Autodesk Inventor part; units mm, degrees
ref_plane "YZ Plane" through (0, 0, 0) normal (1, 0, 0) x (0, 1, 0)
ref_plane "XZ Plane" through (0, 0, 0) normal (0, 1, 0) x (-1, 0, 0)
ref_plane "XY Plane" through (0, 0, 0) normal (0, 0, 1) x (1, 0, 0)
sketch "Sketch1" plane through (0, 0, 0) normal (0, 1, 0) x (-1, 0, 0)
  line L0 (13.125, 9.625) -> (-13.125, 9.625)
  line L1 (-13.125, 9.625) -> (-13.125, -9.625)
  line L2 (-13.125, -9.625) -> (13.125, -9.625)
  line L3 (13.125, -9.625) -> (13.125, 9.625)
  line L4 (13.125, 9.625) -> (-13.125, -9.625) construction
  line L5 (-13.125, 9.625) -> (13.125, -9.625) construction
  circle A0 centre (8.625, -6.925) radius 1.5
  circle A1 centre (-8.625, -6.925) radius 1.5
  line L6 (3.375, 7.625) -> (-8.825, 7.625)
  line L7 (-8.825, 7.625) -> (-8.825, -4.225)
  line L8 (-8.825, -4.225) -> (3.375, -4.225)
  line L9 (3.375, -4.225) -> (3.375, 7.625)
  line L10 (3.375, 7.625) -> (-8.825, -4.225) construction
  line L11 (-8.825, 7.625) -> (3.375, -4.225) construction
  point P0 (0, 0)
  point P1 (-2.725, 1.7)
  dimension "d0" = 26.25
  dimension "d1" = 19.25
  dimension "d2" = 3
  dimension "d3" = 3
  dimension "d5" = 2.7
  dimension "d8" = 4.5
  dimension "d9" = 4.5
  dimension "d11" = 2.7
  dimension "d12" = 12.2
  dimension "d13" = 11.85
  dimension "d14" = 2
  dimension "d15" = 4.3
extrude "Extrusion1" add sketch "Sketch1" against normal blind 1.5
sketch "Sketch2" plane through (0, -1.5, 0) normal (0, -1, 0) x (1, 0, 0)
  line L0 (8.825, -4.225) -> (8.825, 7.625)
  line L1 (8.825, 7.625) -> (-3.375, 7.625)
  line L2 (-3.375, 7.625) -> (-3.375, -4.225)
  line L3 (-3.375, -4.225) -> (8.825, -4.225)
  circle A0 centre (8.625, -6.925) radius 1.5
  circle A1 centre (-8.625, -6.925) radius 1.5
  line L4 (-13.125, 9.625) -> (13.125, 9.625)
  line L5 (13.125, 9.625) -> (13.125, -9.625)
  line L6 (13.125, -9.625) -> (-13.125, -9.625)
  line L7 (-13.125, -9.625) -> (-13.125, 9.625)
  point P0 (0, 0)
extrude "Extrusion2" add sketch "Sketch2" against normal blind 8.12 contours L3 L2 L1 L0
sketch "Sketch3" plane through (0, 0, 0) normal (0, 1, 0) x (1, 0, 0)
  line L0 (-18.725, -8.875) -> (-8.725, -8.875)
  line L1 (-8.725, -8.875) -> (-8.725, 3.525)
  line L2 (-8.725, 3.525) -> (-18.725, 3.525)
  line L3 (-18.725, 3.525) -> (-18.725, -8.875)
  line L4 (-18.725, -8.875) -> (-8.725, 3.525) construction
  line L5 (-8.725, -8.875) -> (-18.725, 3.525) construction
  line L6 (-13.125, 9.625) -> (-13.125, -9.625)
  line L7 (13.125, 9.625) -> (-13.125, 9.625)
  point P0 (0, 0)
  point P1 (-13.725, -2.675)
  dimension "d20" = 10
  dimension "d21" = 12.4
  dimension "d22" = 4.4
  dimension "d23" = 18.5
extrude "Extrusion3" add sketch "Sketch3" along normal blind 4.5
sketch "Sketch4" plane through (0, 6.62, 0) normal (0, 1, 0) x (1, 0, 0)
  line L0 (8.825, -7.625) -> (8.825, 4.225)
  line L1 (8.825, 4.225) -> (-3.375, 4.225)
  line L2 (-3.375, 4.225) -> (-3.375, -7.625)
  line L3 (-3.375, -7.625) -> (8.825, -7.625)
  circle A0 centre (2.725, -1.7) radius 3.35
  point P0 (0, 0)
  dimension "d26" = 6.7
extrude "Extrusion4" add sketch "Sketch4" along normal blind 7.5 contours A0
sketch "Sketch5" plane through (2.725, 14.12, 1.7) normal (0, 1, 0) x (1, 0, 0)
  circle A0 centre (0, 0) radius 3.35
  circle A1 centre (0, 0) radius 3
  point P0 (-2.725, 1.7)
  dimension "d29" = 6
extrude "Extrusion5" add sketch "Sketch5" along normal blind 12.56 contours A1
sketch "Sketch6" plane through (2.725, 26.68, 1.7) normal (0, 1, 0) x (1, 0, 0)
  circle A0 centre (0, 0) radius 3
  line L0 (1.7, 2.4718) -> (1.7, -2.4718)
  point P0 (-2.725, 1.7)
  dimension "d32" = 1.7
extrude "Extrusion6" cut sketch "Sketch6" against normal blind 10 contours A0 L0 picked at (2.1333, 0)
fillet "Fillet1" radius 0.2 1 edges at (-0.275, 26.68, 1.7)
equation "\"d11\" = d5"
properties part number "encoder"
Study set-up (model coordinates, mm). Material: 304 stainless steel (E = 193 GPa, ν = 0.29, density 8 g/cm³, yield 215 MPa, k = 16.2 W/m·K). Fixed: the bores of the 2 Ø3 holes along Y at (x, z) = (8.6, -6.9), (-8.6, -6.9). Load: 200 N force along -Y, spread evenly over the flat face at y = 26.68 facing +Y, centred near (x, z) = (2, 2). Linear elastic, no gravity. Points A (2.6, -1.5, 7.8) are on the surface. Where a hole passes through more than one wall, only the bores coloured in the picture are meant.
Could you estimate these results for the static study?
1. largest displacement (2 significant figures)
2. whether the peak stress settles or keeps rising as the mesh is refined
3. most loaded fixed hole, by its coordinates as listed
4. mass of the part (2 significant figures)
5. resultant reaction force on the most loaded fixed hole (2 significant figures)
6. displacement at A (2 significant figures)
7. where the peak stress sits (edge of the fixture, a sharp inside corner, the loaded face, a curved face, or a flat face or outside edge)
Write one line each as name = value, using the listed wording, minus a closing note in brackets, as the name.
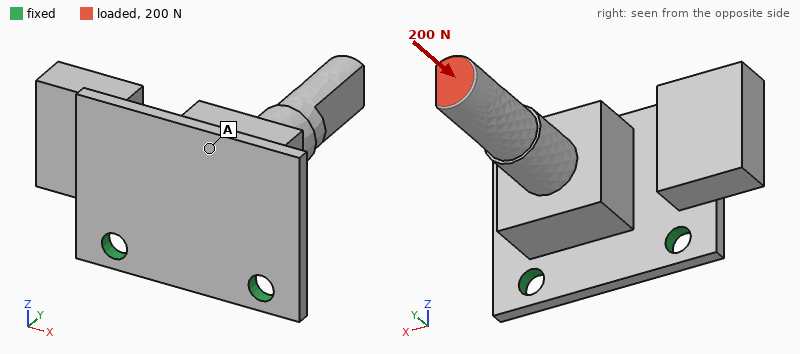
largest displacement = 97 µm
whether the peak stress settles or keeps rising as the mesh is refined = keeps rising
most loaded fixed hole, by its coordinates as listed = (8.6, -6.9)
mass of the part = 23 g
resultant reaction force on the most loaded fixed hole = 120 N
displacement at A = 44 µm
where the peak stress sits = edge of the fixture
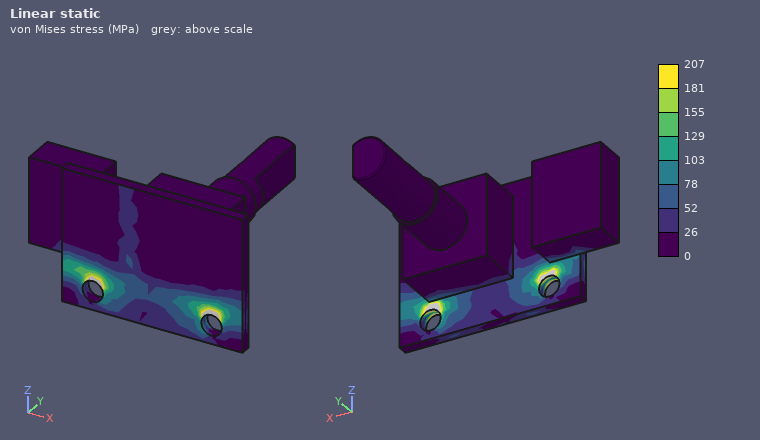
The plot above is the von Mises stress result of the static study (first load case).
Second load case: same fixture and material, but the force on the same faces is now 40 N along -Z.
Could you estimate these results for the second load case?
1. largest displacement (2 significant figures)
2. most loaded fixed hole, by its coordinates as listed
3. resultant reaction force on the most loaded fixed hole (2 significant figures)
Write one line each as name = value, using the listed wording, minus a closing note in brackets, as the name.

largest displacement = 90 µm
most loaded fixed hole, by its coordinates as listed = (8.6, -6.9)
resultant reaction force on the most loaded fixed hole = 32 N
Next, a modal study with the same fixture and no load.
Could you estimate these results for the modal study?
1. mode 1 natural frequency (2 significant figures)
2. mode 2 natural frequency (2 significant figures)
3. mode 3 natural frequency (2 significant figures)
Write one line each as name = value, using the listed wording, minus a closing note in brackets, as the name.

mode 1 natural frequency = 1900 Hz
mode 2 natural frequency = 4800 Hz
mode 3 natural frequency = 5800 Hz
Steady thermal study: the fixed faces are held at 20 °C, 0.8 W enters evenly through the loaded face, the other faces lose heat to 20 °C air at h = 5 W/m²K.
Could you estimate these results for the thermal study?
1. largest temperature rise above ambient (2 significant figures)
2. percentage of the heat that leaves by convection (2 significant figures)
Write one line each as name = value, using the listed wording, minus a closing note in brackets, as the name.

largest temperature rise above ambient = 47 K
percentage of the heat that leaves by convection = 13 %
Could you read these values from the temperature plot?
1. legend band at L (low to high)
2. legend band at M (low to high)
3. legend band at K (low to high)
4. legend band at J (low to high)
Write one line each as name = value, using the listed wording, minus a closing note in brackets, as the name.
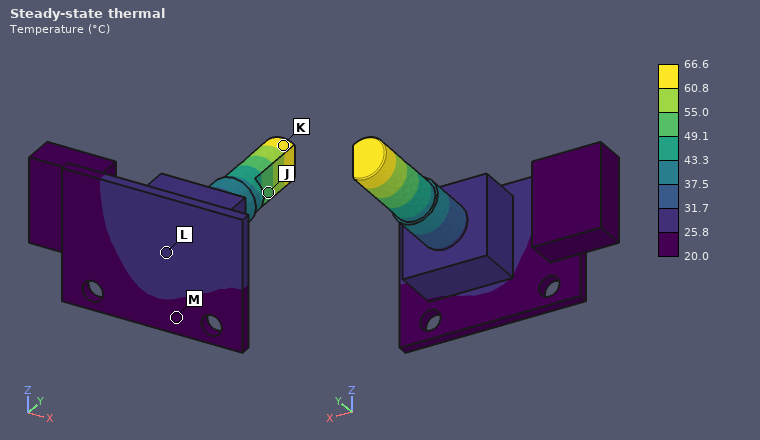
legend band at L = 25.8 to 31.7 °C
legend band at M = 20.0 to 25.8 °C
legend band at K = 60.8 to 66.6 °C
legend band at J = 49.1 to 55.0 °C
